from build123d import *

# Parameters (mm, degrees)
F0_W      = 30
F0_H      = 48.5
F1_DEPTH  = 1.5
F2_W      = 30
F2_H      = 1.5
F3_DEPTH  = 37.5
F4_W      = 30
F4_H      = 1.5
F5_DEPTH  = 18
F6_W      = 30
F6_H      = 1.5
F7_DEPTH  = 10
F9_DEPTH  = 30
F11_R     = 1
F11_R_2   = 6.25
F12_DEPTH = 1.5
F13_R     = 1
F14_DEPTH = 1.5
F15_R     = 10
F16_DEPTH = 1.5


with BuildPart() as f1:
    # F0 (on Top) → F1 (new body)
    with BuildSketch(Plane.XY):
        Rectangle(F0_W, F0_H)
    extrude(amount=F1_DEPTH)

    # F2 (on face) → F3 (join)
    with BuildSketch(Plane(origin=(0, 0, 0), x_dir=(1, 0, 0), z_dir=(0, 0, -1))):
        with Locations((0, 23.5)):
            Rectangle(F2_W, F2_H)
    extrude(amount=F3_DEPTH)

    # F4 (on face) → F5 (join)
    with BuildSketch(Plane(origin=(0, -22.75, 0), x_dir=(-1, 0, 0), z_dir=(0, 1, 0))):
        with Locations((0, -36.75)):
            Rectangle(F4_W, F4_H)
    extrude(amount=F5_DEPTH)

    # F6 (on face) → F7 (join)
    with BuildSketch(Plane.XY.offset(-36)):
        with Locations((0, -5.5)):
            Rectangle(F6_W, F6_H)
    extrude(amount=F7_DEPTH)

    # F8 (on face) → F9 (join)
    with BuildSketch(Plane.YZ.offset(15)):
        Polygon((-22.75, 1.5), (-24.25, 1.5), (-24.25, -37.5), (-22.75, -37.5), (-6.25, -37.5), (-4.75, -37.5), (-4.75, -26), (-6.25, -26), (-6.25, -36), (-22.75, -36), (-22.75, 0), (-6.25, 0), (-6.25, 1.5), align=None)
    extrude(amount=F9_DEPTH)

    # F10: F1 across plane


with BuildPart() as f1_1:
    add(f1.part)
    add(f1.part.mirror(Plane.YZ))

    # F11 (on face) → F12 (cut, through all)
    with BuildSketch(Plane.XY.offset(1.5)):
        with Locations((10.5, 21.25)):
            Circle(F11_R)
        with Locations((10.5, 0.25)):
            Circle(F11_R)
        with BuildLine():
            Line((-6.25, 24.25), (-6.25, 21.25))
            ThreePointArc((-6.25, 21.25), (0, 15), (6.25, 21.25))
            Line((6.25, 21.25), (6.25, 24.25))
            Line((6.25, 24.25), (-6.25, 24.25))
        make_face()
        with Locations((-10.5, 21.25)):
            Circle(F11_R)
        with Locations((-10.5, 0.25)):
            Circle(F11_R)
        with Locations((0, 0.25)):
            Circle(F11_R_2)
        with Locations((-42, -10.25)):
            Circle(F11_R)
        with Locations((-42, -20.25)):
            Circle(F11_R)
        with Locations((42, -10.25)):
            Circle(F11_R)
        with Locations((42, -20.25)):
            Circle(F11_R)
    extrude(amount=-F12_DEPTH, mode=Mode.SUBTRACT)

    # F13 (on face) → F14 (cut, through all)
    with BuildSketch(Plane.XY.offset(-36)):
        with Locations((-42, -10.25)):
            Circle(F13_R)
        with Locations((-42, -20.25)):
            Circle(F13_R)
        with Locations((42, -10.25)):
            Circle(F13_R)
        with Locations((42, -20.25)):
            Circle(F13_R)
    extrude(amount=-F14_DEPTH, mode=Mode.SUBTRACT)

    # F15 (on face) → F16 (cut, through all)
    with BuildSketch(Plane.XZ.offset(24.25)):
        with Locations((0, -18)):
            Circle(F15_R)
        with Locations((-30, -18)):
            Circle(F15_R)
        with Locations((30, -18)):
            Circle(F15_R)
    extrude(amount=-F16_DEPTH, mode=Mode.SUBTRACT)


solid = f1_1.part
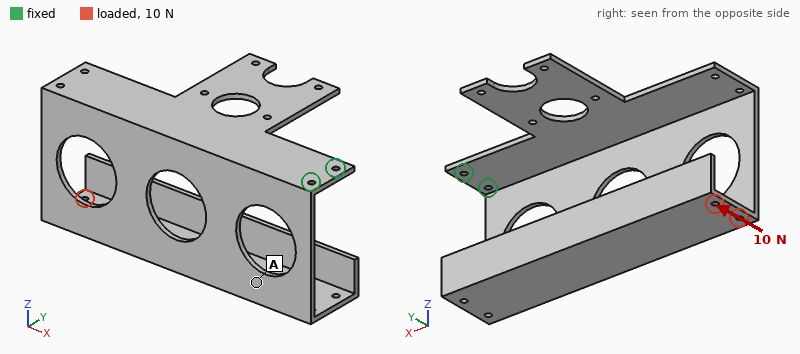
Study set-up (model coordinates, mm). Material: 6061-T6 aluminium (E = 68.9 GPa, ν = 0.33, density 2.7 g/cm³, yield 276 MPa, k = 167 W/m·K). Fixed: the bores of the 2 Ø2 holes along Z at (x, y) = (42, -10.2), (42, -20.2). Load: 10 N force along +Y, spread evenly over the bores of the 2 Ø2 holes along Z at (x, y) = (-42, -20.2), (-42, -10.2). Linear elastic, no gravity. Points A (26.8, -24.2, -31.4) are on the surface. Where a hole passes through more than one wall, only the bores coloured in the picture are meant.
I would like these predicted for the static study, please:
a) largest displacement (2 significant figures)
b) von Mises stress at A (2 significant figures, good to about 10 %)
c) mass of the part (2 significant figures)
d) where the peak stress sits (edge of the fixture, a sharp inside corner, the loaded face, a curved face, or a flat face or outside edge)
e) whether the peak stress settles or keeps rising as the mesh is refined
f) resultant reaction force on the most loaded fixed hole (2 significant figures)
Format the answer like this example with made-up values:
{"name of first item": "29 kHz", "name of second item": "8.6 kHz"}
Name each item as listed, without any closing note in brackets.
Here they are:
{"largest displacement": "1.1 mm", "von Mises stress at A": "5.7 MPa", "mass of the part": "29 g", "where the peak stress sits": "edge of the fixture", "whether the peak stress settles or keeps rising as the mesh is refined": "keeps rising", "resultant reaction force on the most loaded fixed hole": "79 N"}
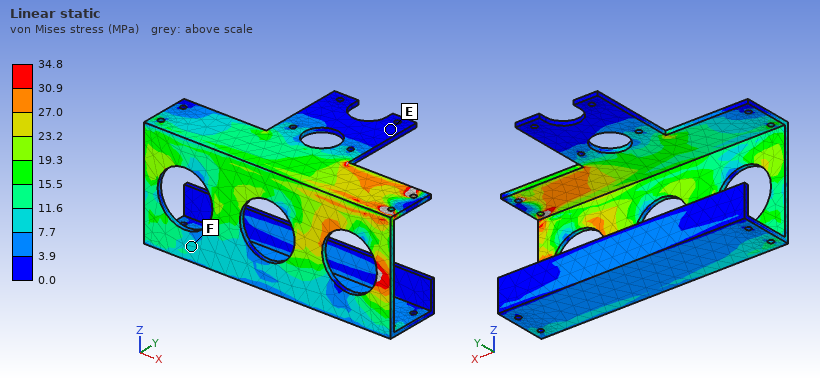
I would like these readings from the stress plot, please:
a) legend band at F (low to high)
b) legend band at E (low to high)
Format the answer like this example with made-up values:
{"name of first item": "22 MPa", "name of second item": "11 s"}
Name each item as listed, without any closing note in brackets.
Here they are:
{"legend band at F": "7.7 to 11.6 MPa", "legend band at E": "0.0 to 3.9 MPa"}
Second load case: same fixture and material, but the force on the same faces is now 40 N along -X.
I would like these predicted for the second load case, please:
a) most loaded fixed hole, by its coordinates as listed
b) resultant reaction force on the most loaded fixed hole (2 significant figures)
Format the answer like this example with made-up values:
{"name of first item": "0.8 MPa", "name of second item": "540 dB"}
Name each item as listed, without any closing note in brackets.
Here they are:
{"most loaded fixed hole, by its coordinates as listed": "(42, -10.2)", "resultant reaction force on the most loaded fixed hole": "29 N"}
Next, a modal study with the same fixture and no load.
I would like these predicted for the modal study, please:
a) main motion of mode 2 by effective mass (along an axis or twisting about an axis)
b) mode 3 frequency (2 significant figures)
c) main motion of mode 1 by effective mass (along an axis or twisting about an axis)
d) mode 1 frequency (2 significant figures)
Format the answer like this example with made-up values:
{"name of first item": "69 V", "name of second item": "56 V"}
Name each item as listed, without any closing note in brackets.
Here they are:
{"main motion of mode 2 by effective mass": "along Z", "mode 3 frequency": "480 Hz", "main motion of mode 1 by effective mass": "along Y", "mode 1 frequency": "170 Hz"}
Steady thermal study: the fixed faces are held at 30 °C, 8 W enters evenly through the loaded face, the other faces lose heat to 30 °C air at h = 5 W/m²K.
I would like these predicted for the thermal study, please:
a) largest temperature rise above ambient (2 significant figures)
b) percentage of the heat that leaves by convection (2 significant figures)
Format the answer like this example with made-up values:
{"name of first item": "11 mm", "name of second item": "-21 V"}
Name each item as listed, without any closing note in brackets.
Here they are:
{"largest temperature rise above ambient": "71 K", "percentage of the heat that leaves by convection": "32 %"}
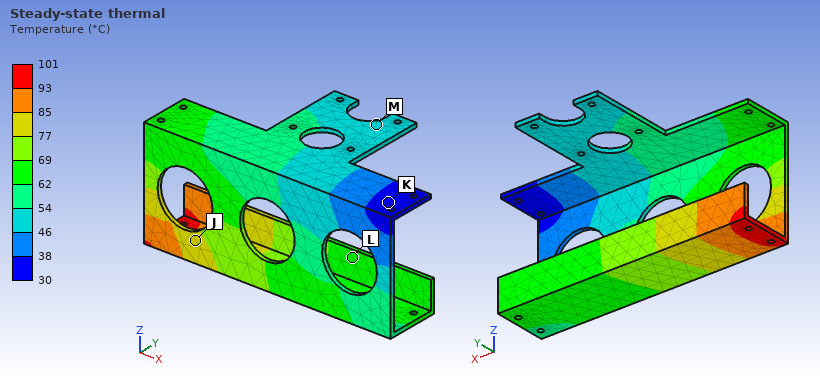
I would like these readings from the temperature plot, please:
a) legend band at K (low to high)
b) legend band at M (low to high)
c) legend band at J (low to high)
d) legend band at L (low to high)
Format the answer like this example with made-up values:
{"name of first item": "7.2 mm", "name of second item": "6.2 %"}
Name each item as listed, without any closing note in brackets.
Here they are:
{"legend band at K": "30 to 38 °C", "legend band at M": "46 to 54 °C", "legend band at J": "77 to 85 °C", "legend band at L": "62 to 69 °C"}
